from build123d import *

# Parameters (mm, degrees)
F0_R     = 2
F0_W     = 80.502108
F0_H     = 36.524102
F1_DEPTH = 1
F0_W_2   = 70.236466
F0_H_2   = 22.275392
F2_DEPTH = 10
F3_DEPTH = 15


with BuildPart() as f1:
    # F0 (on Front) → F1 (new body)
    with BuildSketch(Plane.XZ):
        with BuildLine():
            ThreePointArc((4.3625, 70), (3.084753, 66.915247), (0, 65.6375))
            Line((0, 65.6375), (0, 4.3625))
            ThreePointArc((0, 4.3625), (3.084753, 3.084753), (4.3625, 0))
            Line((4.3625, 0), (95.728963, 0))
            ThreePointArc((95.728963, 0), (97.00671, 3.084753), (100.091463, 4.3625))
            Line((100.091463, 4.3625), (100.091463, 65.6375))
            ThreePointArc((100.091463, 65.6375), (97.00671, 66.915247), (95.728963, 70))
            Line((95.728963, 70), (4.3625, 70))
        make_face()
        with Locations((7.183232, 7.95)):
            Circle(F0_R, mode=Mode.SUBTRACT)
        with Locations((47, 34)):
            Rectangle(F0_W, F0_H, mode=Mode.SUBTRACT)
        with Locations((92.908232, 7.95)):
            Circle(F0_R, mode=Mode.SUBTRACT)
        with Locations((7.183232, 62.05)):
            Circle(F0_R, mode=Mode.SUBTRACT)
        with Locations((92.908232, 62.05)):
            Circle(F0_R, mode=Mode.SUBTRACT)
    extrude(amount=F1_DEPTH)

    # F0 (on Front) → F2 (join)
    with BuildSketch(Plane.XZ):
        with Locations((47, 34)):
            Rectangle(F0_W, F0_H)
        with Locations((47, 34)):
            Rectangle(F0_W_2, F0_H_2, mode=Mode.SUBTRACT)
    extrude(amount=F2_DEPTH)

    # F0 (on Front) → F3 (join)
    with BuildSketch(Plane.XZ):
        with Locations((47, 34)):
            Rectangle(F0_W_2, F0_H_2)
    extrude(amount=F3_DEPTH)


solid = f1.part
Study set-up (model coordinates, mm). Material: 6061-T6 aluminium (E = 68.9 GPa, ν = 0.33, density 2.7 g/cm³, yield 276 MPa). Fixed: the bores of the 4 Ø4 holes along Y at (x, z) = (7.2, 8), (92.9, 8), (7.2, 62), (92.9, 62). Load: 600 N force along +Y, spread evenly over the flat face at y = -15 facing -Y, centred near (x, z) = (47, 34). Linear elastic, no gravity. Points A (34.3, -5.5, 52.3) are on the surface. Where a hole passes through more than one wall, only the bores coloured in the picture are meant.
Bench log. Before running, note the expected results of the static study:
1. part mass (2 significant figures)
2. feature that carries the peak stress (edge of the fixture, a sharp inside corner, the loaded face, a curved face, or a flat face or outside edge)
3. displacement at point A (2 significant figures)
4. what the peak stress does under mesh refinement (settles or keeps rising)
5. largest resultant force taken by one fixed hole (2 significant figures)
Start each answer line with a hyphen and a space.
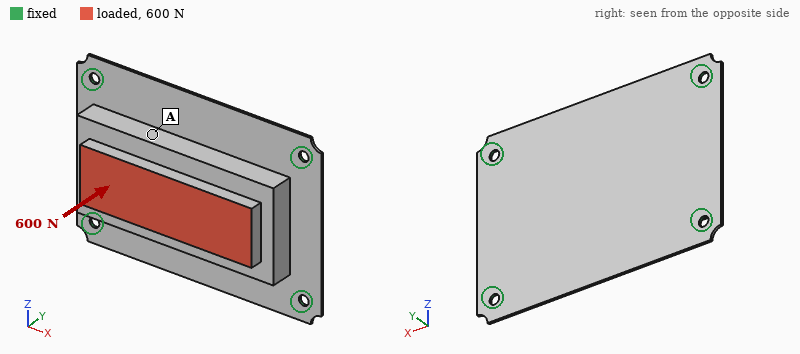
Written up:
- 110 g
- edge of the fixture
- 0.13 mm
- keeps rising
- 220 N
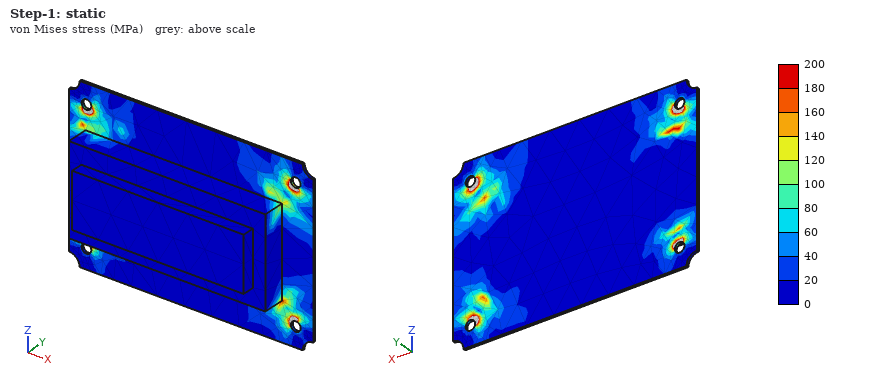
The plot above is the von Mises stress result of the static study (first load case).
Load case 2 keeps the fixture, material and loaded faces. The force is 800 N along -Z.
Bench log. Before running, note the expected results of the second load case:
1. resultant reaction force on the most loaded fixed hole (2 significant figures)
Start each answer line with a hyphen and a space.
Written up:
- 300 N
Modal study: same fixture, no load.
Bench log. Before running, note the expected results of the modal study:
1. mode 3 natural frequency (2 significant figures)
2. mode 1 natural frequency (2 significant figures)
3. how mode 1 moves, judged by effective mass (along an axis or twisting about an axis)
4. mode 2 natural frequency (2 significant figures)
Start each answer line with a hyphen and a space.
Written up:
- 2000 Hz
- 1100 Hz
- along Y
- 1900 Hz
